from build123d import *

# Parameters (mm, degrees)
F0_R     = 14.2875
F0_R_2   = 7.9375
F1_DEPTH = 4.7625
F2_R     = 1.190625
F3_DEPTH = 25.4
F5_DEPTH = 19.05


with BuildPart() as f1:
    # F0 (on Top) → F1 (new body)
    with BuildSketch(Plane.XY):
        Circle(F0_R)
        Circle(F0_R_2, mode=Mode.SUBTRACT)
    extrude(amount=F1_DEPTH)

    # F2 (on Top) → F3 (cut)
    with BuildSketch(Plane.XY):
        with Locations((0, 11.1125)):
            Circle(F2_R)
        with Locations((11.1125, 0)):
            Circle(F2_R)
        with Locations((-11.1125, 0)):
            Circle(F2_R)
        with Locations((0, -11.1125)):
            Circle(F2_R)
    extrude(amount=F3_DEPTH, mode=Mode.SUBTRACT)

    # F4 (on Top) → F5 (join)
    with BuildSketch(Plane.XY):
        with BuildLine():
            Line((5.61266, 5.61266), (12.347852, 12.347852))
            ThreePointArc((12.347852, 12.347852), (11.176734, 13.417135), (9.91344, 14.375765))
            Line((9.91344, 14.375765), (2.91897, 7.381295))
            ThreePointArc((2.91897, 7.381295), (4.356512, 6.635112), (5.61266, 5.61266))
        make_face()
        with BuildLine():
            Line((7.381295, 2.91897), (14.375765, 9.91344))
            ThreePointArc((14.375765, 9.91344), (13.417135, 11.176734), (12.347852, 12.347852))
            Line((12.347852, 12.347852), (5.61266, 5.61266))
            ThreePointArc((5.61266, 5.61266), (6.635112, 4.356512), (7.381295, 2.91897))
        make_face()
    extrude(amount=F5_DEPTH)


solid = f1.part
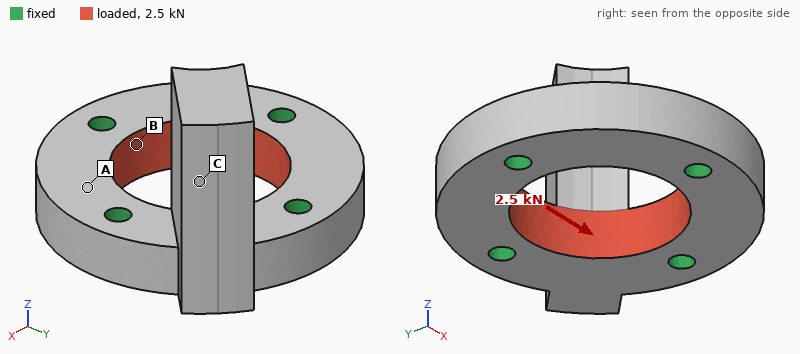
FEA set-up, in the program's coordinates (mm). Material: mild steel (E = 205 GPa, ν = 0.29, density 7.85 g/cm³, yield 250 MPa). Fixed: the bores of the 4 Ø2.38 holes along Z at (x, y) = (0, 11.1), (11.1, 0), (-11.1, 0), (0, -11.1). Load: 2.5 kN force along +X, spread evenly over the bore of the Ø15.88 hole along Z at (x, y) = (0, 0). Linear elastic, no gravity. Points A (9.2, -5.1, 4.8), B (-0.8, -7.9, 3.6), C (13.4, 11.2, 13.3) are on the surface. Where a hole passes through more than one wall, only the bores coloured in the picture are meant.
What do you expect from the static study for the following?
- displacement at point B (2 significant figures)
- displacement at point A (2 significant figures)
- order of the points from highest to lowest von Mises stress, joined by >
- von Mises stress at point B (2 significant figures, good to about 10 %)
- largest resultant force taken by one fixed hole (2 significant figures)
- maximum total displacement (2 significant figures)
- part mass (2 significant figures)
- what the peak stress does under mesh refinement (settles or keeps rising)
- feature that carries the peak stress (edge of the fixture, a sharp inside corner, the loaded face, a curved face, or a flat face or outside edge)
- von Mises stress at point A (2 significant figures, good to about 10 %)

0.55 µm
0.58 µm
B > A > C
18 MPa
710 N
0.78 µm
23 g
keeps rising
edge of the fixture
11 MPa
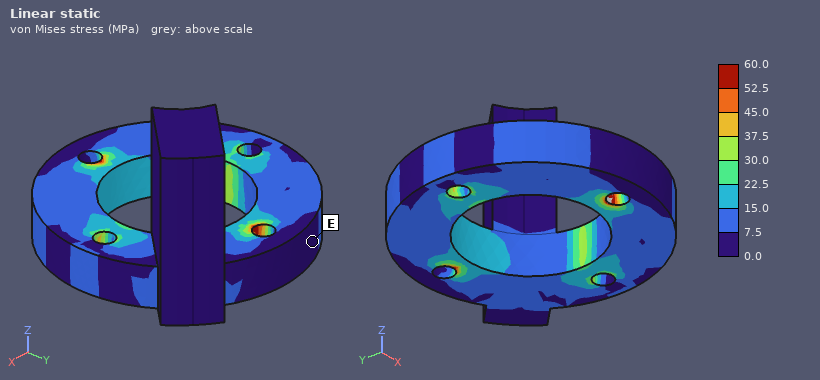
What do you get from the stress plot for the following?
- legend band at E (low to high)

0.0 to 7.5 MPa
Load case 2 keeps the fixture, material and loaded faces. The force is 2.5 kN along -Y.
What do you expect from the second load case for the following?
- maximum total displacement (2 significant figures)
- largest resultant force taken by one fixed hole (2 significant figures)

0.77 µm
710 N
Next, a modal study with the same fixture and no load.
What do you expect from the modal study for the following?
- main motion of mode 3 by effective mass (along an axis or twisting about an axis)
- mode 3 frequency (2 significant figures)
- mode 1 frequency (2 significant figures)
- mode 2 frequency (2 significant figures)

along Z
32 kHz
9200 Hz
15 kHz
